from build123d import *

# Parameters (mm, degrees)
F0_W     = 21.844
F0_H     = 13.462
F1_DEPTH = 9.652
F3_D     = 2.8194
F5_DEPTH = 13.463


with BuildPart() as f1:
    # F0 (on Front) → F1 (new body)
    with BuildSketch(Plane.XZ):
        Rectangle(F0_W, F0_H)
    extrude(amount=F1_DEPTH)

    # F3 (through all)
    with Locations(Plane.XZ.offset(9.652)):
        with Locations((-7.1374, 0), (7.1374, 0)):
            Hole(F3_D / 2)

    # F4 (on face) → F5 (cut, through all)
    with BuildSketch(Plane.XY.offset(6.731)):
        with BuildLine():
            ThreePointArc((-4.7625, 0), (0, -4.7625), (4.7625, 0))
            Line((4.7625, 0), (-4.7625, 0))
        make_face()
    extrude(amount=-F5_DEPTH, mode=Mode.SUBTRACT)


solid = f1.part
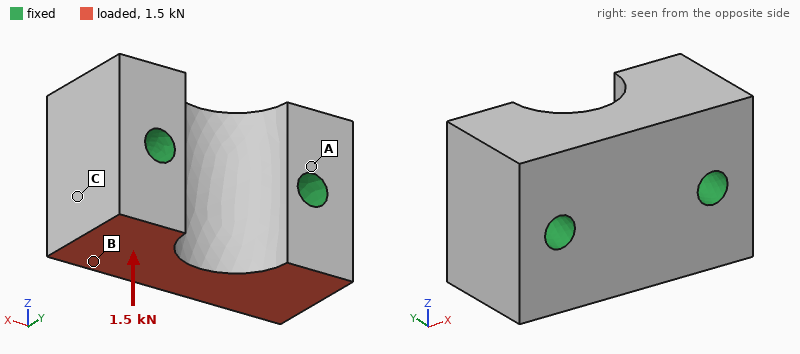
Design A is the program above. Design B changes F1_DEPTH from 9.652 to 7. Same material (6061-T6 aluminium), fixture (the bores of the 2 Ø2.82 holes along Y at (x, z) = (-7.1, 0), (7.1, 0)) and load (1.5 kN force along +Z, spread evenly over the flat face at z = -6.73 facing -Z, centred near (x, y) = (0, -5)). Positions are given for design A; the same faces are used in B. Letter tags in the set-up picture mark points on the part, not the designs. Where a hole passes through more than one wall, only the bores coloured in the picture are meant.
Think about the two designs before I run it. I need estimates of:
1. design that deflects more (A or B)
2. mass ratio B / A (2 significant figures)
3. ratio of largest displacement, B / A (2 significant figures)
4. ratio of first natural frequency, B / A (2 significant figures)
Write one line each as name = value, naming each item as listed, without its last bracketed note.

design that deflects more = B
mass ratio B / A = 0.67
ratio of largest displacement, B / A = 1.5
ratio of first natural frequency, B / A = 0.92
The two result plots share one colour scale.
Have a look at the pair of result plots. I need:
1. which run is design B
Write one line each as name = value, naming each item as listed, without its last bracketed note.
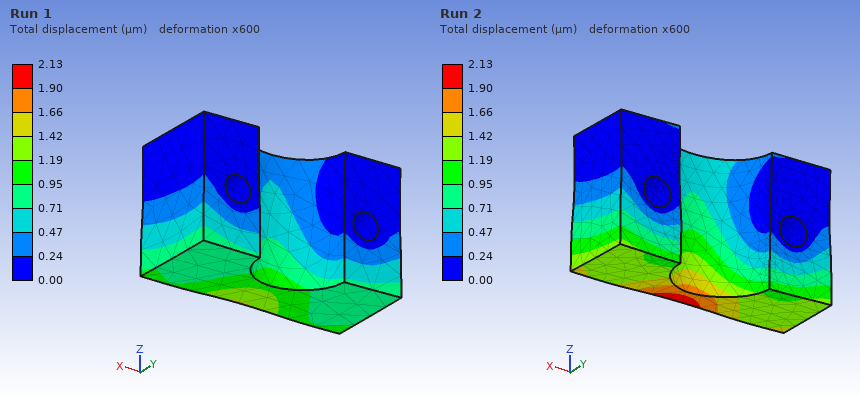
which run is design B = Run 2
